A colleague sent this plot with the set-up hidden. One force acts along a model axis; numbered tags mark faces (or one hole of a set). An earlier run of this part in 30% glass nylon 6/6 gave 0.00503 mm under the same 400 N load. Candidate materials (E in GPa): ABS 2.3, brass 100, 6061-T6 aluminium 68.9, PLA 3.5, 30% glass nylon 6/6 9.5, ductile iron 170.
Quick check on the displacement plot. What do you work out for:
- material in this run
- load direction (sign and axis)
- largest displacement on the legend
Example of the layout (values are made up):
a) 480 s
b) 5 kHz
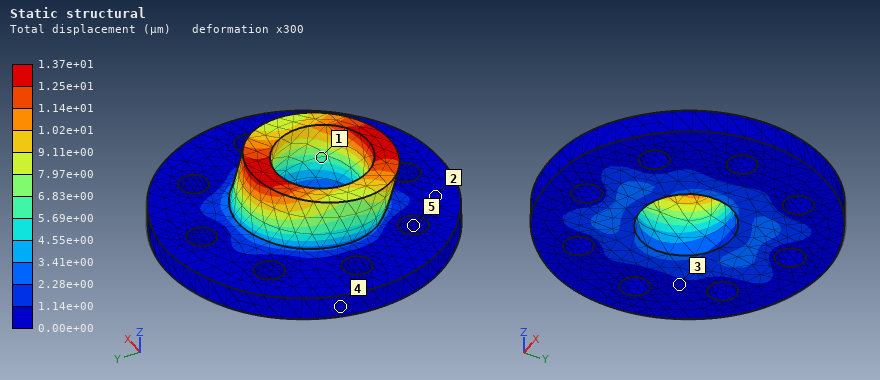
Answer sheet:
a) PLA
b) -Y
c) 1.37e+01 µm
